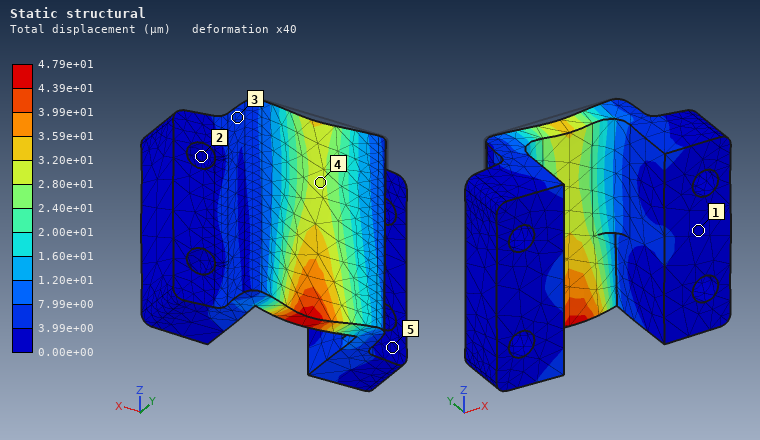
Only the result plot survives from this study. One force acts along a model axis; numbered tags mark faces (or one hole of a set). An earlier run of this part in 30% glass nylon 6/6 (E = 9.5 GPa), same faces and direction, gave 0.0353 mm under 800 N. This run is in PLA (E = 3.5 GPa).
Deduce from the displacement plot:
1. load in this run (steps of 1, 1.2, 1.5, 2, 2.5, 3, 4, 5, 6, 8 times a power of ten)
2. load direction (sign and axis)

400 N
-Y
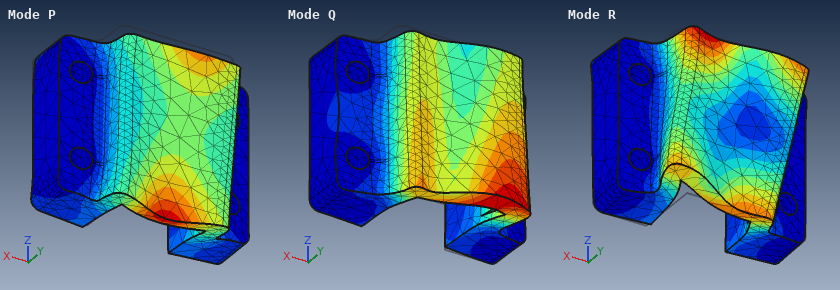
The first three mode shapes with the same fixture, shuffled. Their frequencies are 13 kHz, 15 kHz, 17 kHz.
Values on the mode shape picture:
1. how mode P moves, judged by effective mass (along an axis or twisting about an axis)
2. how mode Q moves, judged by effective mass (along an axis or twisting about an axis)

along Z
along X
